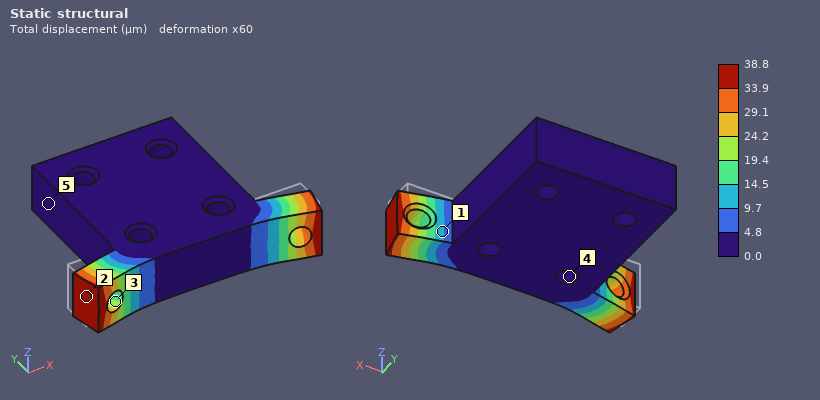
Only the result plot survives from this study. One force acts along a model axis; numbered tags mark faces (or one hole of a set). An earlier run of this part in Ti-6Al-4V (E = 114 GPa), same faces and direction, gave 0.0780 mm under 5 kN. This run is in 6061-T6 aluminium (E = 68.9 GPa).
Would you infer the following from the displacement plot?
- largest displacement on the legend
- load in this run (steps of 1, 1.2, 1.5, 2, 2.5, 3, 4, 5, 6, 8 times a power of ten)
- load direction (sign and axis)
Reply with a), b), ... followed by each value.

a) 38.8 µm
b) 1.5 kN
c) -Y
